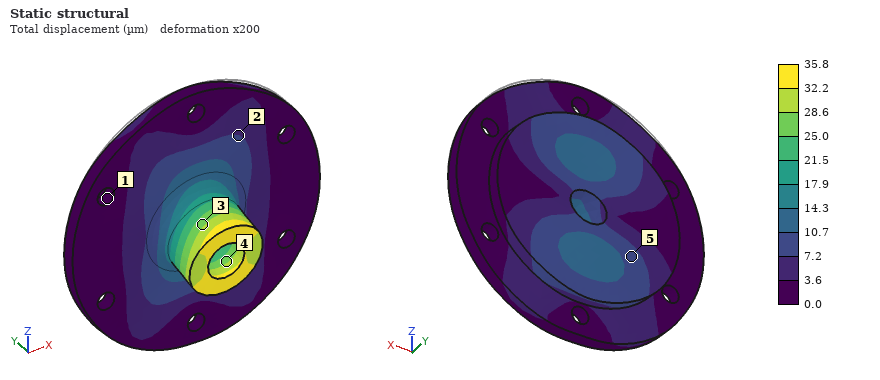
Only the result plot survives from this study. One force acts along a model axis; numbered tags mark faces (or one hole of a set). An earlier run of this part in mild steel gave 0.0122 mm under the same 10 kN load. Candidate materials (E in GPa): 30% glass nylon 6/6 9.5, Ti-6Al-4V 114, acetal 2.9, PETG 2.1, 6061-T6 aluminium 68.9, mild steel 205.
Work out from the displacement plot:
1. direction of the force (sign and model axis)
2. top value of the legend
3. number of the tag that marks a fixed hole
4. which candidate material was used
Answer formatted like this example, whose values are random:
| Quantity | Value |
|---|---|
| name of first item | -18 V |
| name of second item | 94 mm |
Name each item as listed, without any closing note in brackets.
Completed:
| Quantity | Value |
|---|---|
| direction of the force | -Z |
| top value of the legend | 35.8 µm |
| number of the tag that marks a fixed hole | 1 |
| which candidate material was used | 6061-T6 aluminium |
